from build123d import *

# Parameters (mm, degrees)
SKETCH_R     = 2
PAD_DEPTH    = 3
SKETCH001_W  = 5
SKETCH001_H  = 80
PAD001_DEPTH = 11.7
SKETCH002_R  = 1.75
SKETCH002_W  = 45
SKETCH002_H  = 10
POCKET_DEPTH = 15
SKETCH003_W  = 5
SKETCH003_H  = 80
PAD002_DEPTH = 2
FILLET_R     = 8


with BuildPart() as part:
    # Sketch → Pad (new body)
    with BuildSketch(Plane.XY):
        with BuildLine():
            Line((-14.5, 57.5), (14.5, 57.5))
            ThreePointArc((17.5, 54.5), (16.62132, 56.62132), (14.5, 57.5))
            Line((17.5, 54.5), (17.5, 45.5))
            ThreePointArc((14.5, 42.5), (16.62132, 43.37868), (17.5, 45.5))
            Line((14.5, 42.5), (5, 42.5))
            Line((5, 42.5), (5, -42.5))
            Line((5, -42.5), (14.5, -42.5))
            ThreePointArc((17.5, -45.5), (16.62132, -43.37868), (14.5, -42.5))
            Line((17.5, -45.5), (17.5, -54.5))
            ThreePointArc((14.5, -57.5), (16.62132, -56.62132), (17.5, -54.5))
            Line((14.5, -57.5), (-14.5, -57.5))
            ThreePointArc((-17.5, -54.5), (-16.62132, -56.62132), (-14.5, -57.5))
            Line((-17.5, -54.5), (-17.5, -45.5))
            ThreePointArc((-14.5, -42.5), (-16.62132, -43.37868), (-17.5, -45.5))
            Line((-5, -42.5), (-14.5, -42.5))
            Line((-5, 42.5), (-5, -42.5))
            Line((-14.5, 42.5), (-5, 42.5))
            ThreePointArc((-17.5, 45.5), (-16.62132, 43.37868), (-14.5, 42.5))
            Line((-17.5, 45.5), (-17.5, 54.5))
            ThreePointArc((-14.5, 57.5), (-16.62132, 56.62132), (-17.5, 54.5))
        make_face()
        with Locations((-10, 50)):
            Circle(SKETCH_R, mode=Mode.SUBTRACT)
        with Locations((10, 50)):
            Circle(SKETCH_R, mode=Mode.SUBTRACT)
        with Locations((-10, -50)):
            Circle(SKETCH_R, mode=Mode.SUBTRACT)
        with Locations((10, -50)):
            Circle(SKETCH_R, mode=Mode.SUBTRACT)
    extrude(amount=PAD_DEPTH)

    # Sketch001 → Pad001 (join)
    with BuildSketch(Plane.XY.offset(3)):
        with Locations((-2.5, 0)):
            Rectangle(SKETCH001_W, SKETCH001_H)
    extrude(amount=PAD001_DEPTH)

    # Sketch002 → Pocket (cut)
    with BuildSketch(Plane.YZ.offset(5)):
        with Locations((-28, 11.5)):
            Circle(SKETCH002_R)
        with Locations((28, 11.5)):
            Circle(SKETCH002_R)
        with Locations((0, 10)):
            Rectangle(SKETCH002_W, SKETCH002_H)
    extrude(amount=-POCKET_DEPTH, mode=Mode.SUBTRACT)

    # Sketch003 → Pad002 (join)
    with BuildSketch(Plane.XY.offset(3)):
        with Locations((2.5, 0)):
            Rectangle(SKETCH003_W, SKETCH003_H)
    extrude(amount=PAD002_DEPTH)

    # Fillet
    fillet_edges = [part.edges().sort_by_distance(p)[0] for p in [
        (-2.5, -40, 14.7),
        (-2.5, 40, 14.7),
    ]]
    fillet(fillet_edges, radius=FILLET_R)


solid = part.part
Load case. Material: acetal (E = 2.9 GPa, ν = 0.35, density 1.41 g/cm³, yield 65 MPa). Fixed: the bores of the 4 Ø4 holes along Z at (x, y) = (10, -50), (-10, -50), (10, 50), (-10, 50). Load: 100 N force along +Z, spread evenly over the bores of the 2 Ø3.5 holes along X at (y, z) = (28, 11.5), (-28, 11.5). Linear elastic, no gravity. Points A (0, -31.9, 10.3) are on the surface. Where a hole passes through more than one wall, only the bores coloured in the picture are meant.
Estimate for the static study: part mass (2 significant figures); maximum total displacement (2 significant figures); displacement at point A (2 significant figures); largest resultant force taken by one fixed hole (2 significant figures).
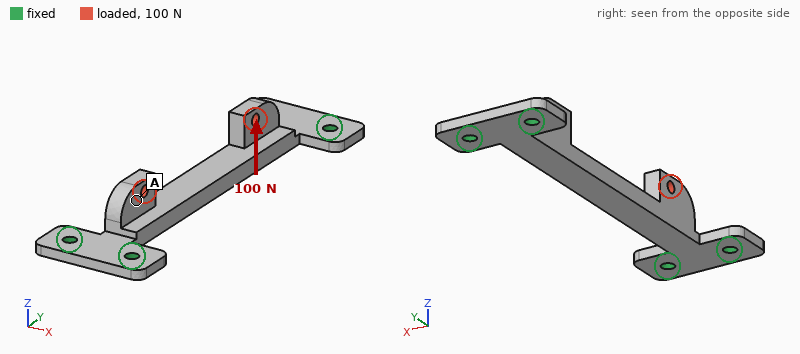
12 g
1.2 mm
0.59 mm
60 N
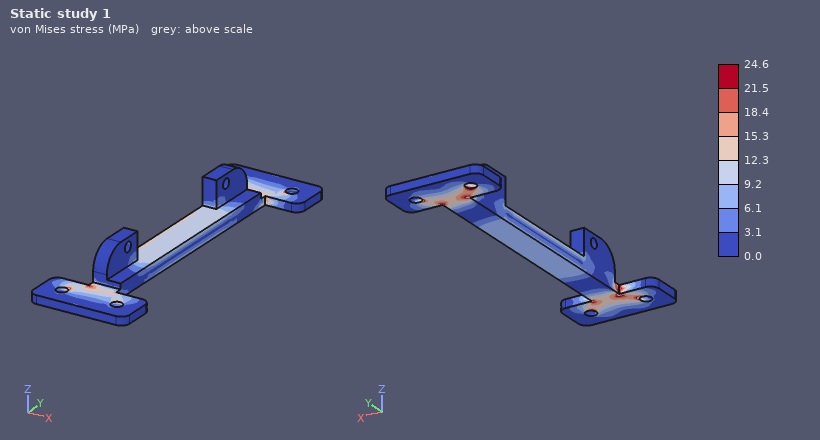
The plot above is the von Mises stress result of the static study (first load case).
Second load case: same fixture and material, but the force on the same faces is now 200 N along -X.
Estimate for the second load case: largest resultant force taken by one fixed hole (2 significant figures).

130 N
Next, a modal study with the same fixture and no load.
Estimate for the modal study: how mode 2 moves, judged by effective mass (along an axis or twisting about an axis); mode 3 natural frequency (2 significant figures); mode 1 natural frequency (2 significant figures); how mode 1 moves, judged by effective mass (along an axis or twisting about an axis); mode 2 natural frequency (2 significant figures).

along X
1500 Hz
540 Hz
along Z
1400 Hz
